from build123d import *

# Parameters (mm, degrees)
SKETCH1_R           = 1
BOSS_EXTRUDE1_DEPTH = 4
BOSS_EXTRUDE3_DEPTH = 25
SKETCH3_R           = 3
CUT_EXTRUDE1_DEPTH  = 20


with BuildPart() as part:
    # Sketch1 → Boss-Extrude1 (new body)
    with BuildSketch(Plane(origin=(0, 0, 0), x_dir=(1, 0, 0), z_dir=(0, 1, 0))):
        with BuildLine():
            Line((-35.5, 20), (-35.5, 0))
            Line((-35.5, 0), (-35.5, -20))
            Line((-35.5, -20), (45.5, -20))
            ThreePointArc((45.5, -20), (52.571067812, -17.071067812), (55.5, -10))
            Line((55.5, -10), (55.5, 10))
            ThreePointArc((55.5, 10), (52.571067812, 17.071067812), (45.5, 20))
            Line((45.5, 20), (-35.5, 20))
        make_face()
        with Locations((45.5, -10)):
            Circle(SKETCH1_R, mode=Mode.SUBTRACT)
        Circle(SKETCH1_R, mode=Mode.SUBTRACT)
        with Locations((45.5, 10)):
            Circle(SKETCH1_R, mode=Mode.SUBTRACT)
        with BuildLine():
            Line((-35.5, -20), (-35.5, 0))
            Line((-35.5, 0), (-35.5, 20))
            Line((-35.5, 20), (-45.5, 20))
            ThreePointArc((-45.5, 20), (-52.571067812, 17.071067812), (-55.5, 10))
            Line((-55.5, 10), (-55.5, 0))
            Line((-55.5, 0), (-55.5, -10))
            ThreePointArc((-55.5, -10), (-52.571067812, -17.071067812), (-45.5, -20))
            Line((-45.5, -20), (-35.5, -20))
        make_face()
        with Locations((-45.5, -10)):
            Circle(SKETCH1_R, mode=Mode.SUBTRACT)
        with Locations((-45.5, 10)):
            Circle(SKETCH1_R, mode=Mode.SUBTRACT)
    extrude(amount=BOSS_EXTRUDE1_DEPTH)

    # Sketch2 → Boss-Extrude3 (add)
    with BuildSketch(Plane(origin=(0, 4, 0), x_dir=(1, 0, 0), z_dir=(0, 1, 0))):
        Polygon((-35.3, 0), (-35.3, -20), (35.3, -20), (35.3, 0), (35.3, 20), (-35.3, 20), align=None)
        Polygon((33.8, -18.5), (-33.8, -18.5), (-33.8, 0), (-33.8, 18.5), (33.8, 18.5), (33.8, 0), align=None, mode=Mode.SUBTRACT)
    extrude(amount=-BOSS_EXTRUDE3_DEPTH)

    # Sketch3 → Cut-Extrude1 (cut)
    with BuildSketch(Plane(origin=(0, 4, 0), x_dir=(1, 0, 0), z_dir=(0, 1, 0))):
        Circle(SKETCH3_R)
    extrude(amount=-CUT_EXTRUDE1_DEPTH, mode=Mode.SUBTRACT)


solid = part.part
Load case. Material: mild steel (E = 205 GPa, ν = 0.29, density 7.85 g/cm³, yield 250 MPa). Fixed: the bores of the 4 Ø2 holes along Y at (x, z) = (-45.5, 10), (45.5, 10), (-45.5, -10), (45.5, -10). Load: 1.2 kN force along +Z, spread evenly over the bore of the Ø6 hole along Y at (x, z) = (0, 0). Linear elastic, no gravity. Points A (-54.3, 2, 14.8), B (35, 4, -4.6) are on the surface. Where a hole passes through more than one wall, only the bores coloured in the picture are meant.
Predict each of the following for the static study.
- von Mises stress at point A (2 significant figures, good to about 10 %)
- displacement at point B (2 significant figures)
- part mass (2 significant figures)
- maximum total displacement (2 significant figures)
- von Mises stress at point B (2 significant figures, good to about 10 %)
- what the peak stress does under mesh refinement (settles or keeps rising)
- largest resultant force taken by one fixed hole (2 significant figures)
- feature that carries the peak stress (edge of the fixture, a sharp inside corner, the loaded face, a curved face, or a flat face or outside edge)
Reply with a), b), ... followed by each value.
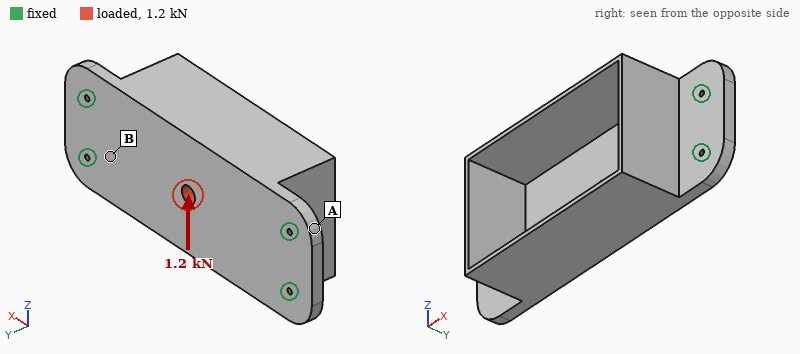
a) 4.0 MPa
b) 1.1 µm
c) 190 g
d) 5.2 µm
e) 9.1 MPa
f) keeps rising
g) 530 N
h) edge of the fixture
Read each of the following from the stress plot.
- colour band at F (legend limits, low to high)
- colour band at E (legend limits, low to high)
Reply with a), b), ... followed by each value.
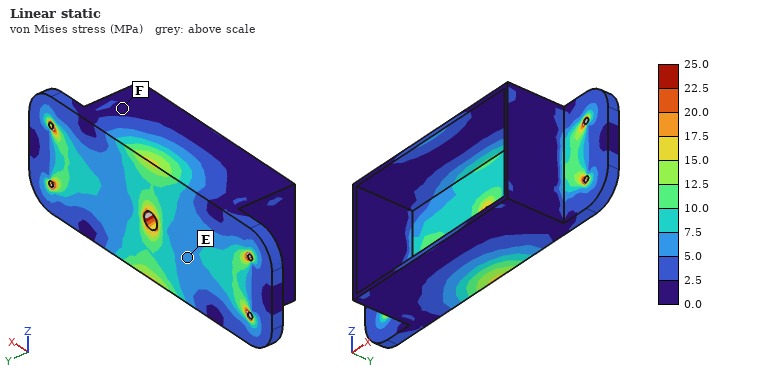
a) 0.0 to 2.5 MPa
b) 5.0 to 7.5 MPa
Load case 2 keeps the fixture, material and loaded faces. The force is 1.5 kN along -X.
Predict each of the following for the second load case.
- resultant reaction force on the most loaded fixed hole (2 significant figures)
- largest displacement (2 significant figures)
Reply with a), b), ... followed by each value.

a) 380 N
b) 1.8 µm
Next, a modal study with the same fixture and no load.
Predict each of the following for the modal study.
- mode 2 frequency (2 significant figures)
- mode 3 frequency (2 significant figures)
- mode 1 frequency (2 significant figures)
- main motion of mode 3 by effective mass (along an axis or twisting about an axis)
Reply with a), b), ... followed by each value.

a) 3500 Hz
b) 4200 Hz
c) 3400 Hz
d) along Y
